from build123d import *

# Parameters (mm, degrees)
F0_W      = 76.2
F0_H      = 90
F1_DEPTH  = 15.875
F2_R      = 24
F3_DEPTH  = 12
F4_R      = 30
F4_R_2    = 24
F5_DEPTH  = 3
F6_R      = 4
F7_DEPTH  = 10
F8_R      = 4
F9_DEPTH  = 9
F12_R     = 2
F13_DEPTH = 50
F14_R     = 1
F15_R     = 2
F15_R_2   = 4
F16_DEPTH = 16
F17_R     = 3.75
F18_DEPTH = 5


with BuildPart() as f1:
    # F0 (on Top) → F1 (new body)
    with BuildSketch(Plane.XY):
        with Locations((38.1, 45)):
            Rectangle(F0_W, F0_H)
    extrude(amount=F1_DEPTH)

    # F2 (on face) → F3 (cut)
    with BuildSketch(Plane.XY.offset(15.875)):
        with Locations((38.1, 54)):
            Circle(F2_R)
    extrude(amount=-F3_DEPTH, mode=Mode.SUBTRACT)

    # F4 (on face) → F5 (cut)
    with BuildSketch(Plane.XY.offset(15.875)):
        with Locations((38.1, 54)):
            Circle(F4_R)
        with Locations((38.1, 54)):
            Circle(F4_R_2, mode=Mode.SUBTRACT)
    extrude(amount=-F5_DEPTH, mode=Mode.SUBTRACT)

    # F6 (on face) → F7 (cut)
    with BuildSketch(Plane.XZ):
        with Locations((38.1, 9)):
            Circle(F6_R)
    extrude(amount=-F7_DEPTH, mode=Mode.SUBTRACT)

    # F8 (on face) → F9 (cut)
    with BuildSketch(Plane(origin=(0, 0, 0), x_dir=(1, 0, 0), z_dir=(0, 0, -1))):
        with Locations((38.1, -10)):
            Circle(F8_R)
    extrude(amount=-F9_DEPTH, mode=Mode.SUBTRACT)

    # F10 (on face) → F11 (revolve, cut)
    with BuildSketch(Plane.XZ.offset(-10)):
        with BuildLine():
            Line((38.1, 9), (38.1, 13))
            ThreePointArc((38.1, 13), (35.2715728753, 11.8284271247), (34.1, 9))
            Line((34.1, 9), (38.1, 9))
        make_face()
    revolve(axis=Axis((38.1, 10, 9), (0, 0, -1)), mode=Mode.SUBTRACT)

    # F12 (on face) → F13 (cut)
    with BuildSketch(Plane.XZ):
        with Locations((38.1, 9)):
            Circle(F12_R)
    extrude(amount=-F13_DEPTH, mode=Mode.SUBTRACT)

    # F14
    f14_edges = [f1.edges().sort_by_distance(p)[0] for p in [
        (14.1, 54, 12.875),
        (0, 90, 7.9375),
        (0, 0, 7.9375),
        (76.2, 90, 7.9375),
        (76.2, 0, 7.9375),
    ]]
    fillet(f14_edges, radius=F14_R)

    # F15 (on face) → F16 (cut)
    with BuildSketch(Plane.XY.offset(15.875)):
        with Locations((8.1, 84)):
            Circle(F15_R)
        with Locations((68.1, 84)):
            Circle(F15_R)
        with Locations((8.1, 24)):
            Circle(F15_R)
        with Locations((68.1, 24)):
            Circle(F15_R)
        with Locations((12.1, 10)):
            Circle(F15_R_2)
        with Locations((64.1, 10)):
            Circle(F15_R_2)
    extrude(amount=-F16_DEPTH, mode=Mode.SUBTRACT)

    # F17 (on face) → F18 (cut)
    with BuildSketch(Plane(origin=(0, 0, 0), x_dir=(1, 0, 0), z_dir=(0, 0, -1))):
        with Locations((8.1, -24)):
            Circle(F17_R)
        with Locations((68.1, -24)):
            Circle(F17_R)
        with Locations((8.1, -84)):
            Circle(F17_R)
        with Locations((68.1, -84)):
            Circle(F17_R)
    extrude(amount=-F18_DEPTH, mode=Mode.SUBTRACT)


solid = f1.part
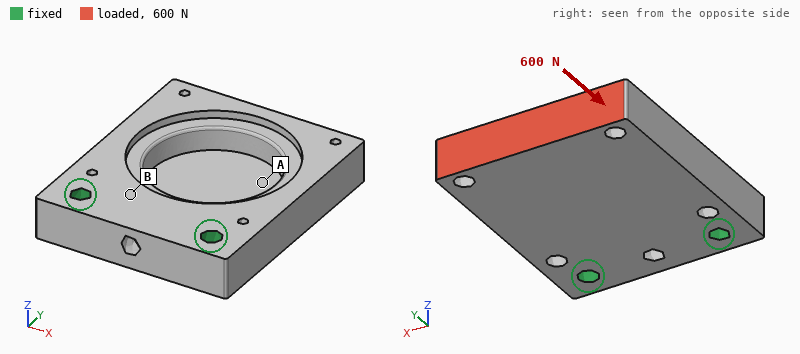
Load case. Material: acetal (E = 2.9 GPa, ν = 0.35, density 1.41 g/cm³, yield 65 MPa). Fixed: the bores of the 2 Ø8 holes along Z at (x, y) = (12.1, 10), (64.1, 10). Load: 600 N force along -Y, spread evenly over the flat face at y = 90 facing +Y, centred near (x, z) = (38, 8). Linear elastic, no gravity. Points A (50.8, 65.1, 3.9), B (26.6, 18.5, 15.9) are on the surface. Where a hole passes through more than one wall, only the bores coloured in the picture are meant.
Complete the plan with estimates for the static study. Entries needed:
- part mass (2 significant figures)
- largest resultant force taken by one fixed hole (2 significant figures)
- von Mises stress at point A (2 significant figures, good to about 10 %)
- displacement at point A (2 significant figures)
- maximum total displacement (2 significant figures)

110 g
300 N
1.6 MPa
0.033 mm
0.12 mm
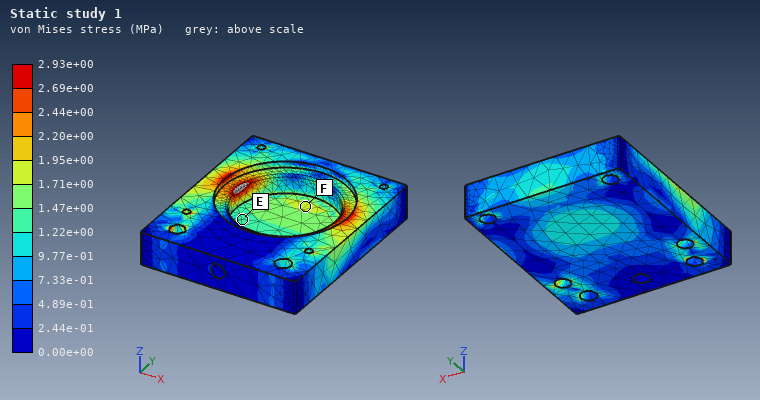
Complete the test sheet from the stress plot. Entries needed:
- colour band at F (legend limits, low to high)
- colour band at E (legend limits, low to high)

1.71e+00 to 1.95e+00 MPa
1.22e+00 to 1.47e+00 MPa
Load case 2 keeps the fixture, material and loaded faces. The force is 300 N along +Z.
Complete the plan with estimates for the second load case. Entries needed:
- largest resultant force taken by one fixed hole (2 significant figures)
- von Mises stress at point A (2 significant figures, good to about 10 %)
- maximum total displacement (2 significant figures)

220 N
2.3 MPa
1.3 mm
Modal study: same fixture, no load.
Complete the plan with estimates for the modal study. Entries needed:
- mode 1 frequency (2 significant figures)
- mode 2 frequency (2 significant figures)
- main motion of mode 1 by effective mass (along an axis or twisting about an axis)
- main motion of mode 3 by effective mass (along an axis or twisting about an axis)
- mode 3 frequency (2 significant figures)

490 Hz
940 Hz
along Z
along X
1600 Hz
